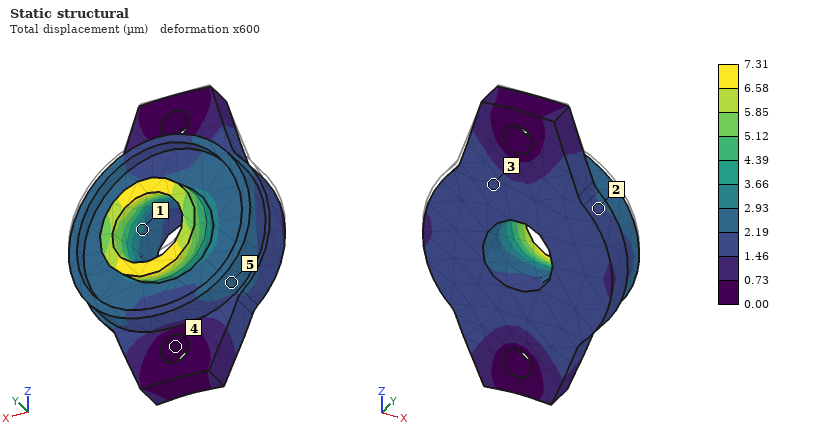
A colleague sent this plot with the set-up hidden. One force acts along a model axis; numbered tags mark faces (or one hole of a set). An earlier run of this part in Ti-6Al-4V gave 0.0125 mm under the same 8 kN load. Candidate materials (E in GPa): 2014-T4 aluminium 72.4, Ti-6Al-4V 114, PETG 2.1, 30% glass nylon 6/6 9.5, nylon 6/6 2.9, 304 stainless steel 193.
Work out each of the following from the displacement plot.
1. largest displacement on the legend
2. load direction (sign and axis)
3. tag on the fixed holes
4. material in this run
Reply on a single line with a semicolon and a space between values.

7.31 µm; -Z; 4; 304 stainless steel
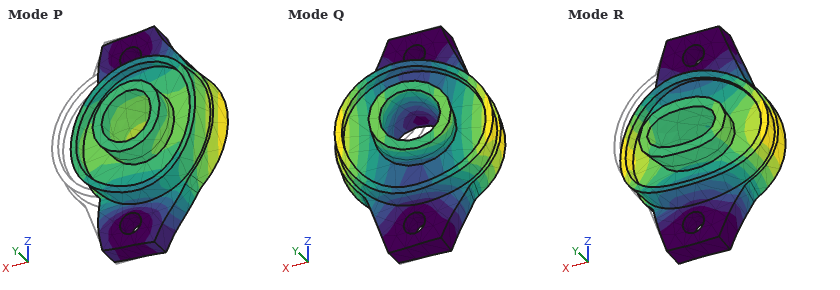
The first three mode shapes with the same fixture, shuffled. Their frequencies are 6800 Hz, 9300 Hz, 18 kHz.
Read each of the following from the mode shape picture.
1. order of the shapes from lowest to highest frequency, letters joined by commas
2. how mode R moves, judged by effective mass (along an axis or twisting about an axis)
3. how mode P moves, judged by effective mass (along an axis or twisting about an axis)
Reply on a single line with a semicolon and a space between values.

Q, R, P; along Y; along X
